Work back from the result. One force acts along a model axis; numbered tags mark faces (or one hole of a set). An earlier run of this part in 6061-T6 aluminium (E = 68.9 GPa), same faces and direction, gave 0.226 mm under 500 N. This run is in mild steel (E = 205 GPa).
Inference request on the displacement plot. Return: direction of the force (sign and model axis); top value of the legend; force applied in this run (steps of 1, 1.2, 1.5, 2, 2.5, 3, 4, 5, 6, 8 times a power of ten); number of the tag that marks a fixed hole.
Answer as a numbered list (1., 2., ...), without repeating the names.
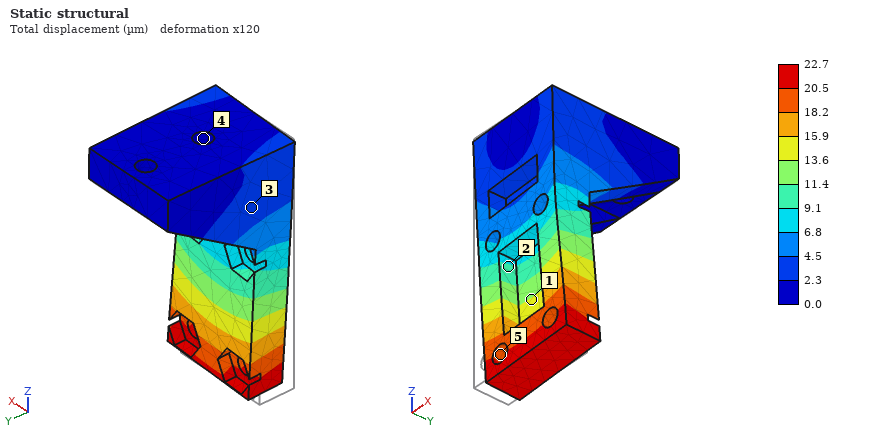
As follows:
1. +X
2. 22.7 µm
3. 150 N
4. 4
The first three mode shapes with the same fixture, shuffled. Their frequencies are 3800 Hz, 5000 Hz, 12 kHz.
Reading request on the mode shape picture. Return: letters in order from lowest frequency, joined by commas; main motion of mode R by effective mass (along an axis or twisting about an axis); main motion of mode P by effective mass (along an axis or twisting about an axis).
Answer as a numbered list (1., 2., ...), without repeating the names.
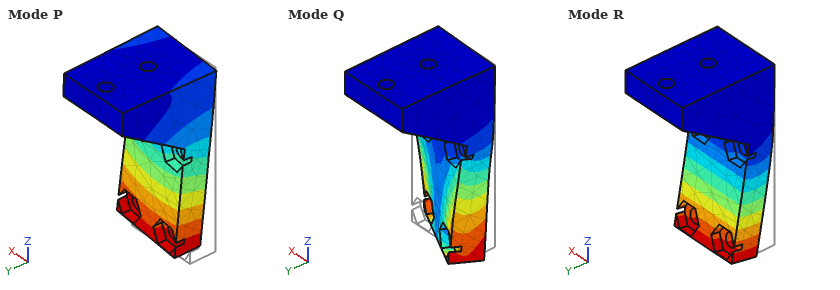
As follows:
1. R, P, Q
2. along Y
3. along X
